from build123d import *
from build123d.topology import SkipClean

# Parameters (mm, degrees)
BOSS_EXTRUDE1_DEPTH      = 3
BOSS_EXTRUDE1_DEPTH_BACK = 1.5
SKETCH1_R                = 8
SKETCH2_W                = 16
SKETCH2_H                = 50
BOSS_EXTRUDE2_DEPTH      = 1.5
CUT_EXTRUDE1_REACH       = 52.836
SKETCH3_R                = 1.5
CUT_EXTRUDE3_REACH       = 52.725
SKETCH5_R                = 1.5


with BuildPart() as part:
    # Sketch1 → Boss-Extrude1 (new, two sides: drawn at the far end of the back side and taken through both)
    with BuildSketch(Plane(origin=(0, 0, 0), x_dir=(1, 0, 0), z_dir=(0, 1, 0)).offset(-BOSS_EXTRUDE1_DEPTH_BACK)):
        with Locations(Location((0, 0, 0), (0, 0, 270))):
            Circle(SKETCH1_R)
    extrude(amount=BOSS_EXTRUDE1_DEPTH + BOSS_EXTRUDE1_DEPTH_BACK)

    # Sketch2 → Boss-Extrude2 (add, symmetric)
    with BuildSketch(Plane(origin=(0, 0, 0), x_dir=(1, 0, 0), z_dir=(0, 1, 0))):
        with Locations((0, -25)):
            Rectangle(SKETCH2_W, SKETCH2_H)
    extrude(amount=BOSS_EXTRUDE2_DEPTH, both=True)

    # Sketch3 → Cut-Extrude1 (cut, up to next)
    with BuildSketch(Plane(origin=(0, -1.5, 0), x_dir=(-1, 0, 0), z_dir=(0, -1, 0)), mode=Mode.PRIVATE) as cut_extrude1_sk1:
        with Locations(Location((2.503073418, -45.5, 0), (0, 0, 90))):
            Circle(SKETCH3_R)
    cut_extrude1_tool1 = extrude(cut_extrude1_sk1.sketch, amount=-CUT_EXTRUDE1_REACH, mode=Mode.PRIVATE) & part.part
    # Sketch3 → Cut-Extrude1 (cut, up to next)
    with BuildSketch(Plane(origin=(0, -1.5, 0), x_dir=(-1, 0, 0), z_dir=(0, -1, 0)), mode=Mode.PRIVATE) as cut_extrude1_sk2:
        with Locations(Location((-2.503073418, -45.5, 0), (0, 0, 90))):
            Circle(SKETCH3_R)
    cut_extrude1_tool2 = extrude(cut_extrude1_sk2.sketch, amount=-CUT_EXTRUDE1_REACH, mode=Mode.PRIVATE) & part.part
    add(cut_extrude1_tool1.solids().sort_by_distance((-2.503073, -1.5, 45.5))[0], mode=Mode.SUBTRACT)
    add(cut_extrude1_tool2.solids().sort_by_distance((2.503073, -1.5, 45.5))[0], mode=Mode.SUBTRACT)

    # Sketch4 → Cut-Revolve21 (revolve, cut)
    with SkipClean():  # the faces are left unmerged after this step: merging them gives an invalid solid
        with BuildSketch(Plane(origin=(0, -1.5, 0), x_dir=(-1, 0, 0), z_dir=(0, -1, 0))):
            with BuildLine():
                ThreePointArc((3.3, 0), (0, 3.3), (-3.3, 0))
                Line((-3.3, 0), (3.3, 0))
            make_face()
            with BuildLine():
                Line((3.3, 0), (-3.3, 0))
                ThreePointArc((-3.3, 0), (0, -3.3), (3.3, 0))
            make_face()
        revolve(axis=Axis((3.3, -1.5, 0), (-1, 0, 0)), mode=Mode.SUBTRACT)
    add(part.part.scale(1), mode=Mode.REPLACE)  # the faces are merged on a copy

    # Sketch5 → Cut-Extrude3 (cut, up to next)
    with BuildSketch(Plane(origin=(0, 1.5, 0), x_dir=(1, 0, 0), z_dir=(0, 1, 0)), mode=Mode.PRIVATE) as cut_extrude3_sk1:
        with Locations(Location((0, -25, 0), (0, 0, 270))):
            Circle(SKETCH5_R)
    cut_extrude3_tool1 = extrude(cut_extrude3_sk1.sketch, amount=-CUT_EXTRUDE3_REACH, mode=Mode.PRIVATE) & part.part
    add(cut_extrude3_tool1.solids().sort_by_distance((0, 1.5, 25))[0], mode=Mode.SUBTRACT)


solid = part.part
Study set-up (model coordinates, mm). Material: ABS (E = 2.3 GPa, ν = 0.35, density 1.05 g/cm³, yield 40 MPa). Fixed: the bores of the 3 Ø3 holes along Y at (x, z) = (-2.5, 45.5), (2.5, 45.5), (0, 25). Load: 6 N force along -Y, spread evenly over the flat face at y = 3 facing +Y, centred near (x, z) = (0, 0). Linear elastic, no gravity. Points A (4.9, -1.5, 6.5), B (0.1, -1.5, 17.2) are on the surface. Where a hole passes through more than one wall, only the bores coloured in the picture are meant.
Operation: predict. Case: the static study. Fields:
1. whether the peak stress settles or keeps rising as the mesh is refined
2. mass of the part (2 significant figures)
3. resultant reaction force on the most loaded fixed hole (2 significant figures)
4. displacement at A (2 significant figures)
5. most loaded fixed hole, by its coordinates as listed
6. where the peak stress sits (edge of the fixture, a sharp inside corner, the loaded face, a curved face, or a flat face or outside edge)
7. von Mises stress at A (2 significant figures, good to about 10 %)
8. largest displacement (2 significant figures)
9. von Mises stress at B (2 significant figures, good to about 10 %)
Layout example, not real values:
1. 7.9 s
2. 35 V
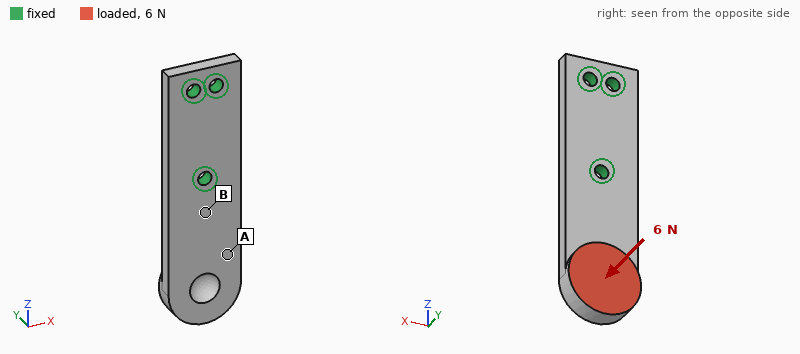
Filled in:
1. keeps rising
2. 3.0 g
3. 7.6 N
4. 0.23 mm
5. (0, 25)
6. edge of the fixture
7. 1.4 MPa
8. 0.54 mm
9. 3.9 MPa
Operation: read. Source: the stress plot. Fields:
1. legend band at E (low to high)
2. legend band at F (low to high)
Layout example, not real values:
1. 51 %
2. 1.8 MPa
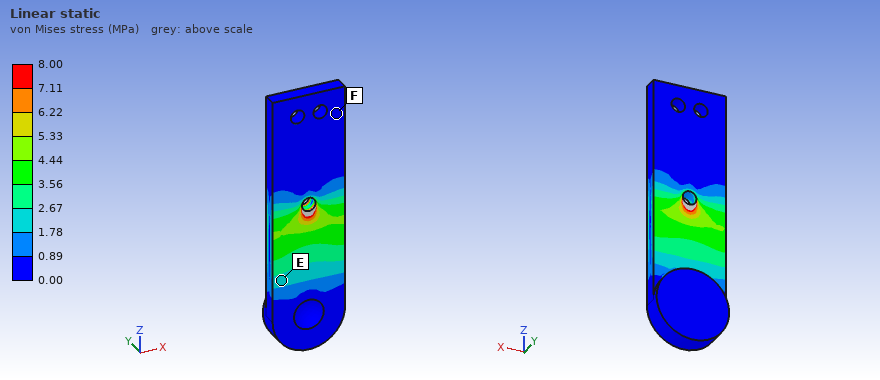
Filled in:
1. 1.78 to 2.67 MPa
2. 0.00 to 0.89 MPa
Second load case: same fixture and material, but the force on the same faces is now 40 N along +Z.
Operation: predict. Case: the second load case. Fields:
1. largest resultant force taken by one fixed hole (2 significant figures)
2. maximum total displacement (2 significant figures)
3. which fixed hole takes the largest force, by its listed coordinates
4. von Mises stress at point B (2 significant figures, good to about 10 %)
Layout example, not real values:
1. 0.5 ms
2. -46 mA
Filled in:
1. 33 N
2. 0.66 mm
3. (0, 25)
4. 3.6 MPa
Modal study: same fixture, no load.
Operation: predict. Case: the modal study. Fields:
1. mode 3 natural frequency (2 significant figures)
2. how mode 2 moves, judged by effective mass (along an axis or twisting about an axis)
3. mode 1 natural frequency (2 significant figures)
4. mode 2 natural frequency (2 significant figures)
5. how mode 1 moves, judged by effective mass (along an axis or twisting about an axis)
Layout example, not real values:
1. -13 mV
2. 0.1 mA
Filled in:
1. 2500 Hz
2. along X
3. 640 Hz
4. 2100 Hz
5. along Y
